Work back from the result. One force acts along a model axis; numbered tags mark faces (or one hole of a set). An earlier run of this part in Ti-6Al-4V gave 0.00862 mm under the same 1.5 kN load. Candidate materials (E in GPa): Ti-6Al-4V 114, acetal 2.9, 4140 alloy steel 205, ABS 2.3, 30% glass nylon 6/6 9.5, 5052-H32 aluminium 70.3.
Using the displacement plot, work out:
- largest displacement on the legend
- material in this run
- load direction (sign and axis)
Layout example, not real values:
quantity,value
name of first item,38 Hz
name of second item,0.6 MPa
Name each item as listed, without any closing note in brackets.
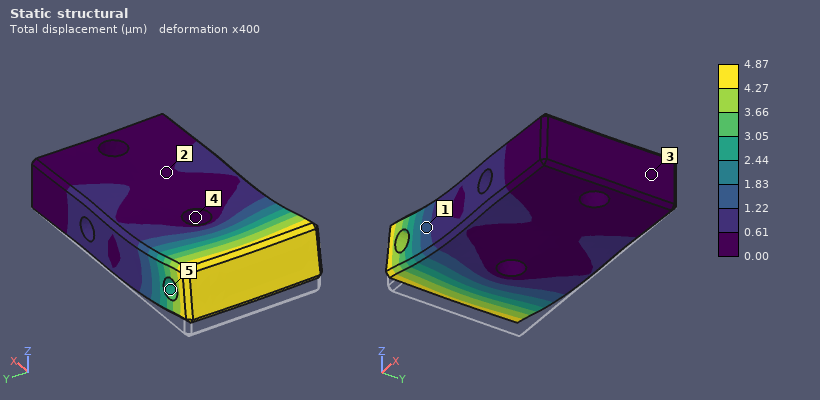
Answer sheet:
quantity,value
largest displacement on the legend,4.87 µm
material in this run,4140 alloy steel
load direction,+Z
